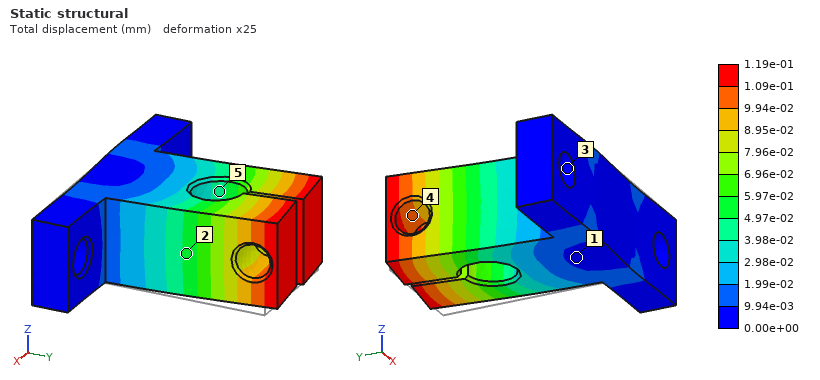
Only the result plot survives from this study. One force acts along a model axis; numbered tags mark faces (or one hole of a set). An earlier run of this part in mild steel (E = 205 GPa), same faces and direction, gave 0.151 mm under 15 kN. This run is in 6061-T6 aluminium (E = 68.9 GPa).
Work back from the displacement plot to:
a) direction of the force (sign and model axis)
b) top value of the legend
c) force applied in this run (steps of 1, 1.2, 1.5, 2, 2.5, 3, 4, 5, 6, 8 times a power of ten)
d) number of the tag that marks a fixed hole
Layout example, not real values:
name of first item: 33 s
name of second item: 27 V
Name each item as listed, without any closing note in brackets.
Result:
direction of the force: -X
top value of the legend: 1.19e-01 mm
force applied in this run: 4 kN
number of the tag that marks a fixed hole: 3
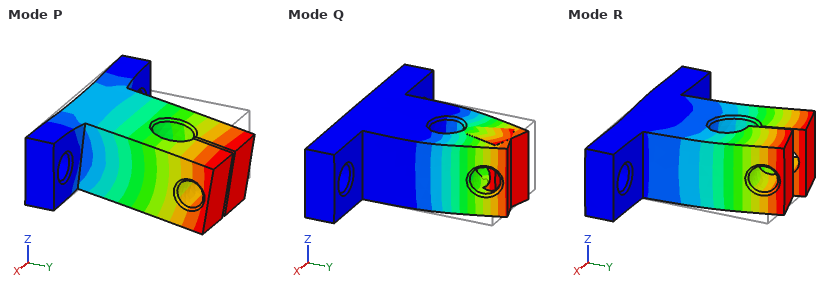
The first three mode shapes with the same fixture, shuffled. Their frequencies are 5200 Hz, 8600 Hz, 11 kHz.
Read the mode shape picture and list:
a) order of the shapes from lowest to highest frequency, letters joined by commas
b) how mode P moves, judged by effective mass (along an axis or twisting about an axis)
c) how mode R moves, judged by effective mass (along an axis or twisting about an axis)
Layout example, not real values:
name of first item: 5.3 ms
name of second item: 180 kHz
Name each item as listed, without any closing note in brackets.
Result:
order of the shapes from lowest to highest frequency, letters joined by commas: P, R, Q
how mode P moves, judged by effective mass: along Z
how mode R moves, judged by effective mass: along X
